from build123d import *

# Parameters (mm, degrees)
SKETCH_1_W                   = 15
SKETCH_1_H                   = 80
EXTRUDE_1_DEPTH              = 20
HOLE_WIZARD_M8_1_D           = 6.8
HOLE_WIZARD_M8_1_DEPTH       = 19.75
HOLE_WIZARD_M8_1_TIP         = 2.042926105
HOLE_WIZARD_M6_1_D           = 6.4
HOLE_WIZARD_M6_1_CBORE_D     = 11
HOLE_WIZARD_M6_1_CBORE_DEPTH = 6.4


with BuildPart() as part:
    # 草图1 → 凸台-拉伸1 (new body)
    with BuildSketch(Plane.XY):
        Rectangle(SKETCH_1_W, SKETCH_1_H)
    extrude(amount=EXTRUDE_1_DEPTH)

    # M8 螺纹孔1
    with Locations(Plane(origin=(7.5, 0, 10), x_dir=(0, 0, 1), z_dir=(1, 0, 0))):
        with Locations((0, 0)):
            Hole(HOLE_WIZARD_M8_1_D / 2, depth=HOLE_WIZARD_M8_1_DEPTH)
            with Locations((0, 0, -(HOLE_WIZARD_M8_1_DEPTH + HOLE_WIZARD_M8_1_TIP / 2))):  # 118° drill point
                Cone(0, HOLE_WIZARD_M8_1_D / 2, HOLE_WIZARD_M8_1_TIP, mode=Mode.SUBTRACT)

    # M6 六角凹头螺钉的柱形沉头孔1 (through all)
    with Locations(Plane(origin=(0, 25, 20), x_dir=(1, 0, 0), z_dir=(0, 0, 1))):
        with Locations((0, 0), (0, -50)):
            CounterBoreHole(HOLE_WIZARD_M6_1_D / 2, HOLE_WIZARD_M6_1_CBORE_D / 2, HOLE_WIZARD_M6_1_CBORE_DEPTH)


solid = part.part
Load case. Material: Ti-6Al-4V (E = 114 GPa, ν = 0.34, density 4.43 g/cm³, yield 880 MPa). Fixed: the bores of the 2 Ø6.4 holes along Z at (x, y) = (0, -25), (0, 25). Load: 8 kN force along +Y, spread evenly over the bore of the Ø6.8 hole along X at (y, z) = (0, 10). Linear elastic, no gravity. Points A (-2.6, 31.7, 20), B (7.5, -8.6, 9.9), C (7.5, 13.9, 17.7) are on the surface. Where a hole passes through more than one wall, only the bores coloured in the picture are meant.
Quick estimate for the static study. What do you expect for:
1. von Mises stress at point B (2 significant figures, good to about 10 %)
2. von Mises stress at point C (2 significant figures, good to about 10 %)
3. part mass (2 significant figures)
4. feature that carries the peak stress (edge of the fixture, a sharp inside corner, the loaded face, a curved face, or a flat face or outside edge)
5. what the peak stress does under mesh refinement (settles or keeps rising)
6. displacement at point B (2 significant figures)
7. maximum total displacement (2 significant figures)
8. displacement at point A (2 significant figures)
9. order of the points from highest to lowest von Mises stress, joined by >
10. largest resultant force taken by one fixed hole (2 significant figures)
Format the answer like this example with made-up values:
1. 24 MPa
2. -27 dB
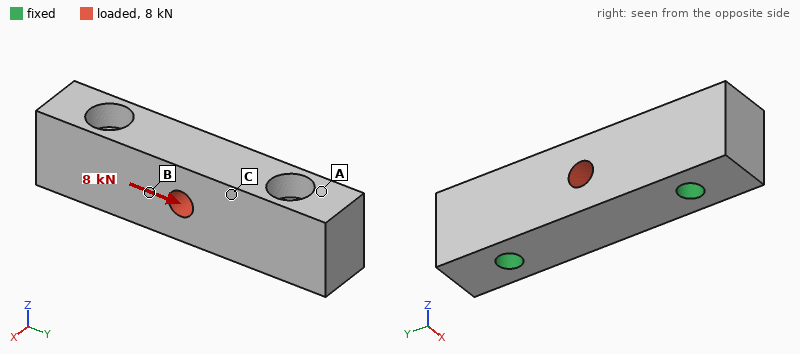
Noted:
1. 23 MPa
2. 8.5 MPa
3. 95 g
4. edge of the fixture
5. keeps rising
6. 2.6 µm
7. 4.1 µm
8. 0.92 µm
9. B > C > A
10. 4.0 kN
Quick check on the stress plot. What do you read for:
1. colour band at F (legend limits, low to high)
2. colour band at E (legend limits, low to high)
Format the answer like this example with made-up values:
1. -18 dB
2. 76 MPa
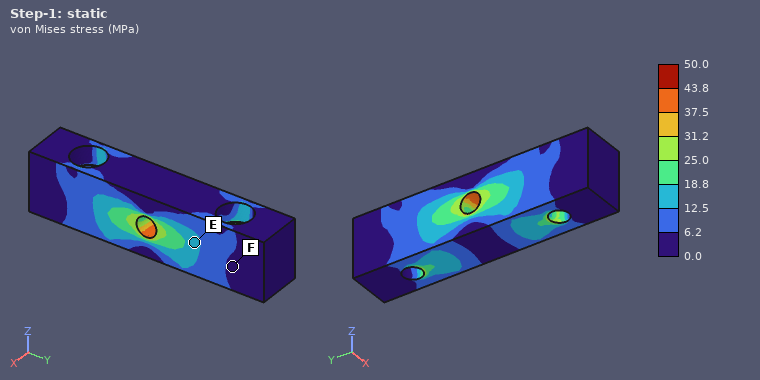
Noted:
1. 0.0 to 6.2 MPa
2. 12.5 to 18.8 MPa
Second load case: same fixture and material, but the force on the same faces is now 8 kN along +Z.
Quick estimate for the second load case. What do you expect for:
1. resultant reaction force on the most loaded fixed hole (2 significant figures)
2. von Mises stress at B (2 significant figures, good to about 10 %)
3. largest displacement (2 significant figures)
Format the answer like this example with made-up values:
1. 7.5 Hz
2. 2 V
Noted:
1. 4.2 kN
2. 34 MPa
3. 15 µm
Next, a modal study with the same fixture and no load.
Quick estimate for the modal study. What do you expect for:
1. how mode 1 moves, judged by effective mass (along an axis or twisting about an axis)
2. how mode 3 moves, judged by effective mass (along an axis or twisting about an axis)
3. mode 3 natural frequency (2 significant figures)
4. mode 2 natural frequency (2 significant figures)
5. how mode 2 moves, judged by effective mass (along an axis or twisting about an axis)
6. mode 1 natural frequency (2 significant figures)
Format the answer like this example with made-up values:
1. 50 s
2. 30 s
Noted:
1. along X
2. twisting about Y
3. 25 kHz
4. 23 kHz
5. along Z
6. 18 kHz
